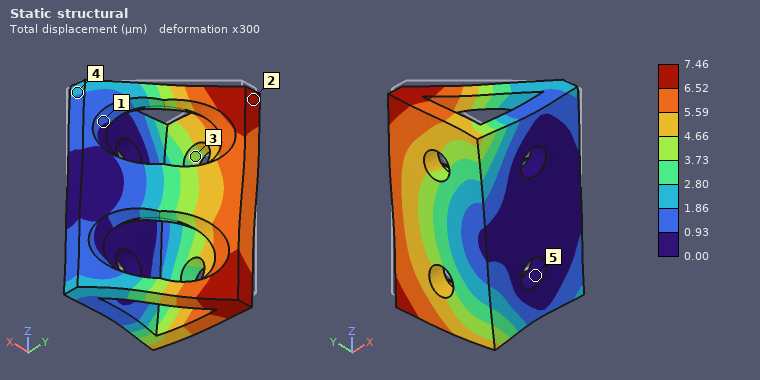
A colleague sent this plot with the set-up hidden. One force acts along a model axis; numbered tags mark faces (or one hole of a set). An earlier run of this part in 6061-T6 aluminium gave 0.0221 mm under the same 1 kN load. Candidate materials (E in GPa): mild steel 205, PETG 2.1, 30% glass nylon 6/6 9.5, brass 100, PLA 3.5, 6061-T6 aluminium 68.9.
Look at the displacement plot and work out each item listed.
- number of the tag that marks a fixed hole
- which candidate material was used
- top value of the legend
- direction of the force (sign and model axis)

5
mild steel
7.46 µm
-Z
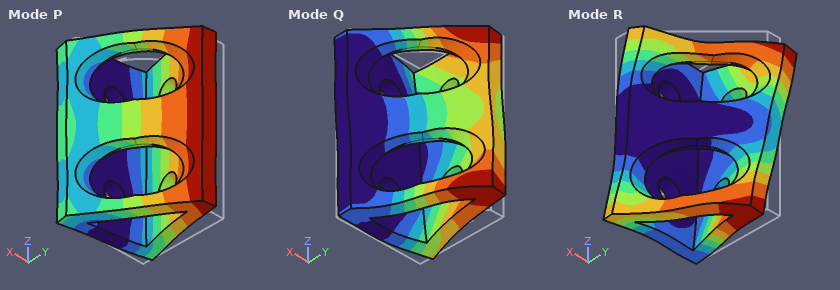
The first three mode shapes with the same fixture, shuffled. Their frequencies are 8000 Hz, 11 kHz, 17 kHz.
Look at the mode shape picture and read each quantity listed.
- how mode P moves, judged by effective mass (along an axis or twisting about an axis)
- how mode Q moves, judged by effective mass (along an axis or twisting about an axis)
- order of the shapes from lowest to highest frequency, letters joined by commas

along X
along Z
P, Q, R
